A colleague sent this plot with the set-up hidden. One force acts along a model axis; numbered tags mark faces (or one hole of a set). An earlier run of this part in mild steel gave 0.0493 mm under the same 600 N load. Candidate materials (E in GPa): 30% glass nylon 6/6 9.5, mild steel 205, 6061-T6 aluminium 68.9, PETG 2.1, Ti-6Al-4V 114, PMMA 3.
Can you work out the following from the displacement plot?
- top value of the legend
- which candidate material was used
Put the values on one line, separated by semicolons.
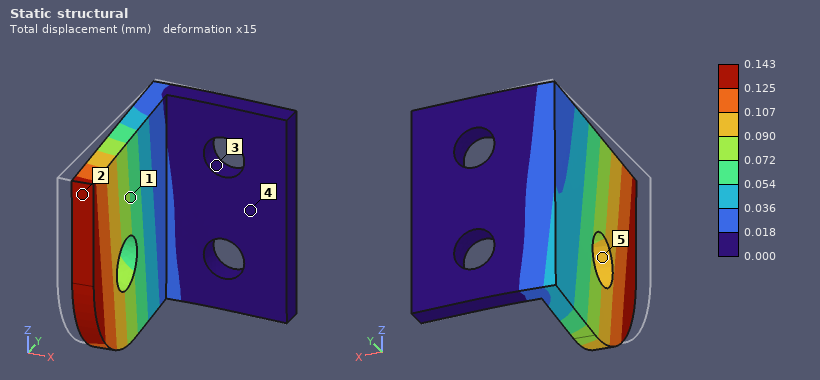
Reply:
0.143 mm; 6061-T6 aluminium
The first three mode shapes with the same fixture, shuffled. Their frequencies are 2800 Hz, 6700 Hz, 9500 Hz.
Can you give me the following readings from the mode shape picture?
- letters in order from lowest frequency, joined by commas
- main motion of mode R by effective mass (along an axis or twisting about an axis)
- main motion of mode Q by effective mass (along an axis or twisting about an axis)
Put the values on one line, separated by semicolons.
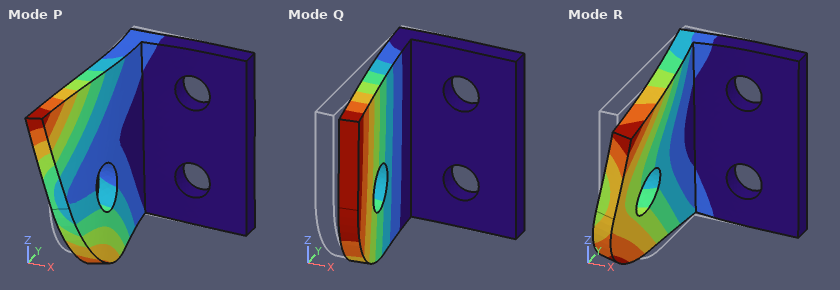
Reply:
Q, R, P; along Z; along X
